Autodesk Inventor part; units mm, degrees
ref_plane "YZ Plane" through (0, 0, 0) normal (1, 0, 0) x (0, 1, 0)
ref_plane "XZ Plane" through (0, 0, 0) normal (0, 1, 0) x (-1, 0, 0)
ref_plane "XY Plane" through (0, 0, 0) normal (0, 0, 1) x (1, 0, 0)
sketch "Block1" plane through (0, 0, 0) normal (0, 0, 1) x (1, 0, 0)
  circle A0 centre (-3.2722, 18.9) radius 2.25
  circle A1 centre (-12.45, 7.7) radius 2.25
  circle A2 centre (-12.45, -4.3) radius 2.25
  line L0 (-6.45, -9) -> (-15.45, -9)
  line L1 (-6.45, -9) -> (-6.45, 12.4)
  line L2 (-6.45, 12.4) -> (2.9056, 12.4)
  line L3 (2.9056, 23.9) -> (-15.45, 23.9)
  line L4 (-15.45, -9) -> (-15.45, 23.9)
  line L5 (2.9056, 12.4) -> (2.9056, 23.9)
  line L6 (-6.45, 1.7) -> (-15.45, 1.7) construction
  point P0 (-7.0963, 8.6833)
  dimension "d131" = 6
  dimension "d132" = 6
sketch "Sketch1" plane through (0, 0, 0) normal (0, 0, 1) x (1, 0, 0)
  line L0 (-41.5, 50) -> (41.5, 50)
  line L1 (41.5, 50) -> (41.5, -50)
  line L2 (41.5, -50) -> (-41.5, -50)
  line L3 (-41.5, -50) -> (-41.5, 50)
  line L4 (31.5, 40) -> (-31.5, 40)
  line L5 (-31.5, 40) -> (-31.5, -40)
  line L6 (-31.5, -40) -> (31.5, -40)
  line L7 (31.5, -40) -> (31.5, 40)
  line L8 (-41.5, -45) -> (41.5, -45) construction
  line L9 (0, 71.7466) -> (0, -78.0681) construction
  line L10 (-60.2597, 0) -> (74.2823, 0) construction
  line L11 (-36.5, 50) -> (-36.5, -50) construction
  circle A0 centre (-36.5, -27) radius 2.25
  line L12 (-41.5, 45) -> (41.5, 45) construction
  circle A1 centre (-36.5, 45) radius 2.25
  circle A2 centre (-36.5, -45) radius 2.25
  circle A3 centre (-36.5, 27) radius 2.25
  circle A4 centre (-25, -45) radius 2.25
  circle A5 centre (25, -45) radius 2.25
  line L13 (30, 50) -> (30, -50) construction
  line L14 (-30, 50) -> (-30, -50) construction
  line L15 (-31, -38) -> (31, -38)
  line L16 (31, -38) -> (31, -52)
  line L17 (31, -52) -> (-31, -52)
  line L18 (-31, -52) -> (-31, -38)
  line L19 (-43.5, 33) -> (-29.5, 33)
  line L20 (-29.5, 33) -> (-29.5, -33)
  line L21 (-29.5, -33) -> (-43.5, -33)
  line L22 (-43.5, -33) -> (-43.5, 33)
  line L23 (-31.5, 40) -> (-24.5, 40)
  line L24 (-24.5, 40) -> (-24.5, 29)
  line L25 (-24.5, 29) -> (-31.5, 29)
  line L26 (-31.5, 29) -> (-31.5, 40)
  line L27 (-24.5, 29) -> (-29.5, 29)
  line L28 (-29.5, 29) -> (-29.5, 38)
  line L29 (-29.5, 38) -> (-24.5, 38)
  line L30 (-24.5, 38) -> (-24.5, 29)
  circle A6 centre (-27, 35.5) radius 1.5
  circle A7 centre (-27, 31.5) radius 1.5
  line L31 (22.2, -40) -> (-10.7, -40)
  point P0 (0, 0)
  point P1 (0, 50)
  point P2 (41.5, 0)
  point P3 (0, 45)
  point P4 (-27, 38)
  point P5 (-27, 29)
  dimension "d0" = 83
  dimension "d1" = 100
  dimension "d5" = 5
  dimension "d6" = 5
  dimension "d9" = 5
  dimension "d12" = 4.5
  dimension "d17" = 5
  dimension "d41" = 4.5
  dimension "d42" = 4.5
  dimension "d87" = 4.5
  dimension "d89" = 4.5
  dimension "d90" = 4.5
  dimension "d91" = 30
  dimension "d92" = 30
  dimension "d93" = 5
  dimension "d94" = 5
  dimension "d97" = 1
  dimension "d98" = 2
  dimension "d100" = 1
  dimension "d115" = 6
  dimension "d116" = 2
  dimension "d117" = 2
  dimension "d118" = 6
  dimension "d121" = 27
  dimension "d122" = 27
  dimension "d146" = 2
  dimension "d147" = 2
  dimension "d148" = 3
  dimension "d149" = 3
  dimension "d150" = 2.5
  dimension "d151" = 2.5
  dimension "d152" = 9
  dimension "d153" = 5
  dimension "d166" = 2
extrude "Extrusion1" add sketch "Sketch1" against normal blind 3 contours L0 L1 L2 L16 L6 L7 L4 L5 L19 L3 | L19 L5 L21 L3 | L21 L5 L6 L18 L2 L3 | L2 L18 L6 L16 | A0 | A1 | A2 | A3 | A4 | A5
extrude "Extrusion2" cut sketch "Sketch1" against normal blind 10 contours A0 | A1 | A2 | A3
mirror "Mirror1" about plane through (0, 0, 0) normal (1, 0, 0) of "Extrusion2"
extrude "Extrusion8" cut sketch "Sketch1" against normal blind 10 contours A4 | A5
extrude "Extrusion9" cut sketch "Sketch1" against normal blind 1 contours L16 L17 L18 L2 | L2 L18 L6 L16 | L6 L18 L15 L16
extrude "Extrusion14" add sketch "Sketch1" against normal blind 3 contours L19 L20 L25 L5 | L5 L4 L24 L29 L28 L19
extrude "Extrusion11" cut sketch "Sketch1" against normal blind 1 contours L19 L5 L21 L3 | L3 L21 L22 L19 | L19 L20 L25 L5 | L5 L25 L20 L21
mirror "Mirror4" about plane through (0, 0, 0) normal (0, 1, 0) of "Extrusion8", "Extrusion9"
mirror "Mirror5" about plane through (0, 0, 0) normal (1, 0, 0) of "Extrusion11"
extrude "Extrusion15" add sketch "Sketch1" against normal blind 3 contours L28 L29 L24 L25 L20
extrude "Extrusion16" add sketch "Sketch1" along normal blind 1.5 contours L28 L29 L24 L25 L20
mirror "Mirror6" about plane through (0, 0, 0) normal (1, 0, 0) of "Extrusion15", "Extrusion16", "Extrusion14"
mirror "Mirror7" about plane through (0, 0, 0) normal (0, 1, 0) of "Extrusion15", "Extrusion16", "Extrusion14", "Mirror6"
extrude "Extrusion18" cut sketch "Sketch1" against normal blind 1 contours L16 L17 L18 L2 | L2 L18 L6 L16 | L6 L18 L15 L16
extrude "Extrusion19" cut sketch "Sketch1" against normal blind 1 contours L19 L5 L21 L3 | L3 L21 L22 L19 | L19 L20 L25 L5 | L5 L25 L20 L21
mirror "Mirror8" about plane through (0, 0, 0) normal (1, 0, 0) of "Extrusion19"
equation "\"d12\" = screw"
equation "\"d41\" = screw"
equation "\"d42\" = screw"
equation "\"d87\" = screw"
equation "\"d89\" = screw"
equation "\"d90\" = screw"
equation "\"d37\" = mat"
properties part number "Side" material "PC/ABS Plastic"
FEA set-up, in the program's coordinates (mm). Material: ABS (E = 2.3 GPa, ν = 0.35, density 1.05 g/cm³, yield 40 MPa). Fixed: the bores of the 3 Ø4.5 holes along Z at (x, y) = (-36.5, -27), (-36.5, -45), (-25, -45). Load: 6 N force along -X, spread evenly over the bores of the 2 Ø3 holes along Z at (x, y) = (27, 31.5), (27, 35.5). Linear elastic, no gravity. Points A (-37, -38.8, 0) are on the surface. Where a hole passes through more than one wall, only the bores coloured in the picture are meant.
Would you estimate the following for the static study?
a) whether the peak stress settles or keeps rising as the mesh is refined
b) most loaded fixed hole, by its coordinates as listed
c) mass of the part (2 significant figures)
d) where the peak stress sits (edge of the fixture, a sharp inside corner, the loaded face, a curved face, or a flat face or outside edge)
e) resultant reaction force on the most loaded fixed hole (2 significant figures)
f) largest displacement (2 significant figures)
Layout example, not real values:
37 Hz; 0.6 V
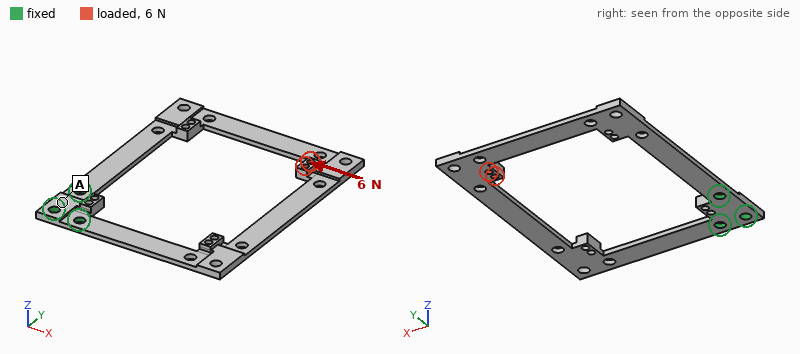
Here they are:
keeps rising; (-36.5, -27); 8.0 g; edge of the fixture; 9.8 N; 1.6 mm
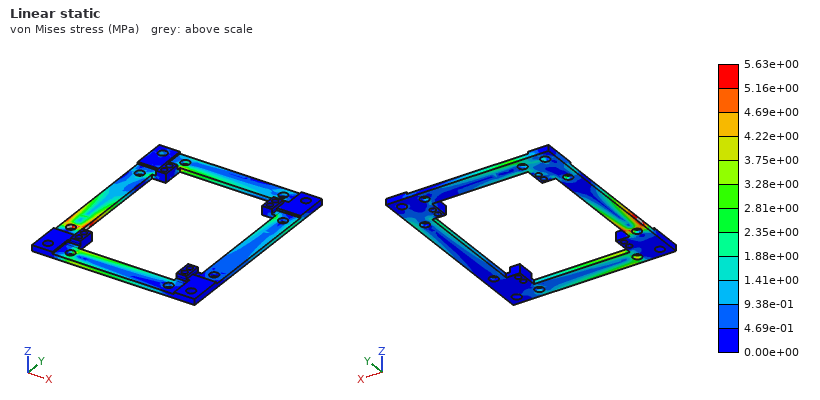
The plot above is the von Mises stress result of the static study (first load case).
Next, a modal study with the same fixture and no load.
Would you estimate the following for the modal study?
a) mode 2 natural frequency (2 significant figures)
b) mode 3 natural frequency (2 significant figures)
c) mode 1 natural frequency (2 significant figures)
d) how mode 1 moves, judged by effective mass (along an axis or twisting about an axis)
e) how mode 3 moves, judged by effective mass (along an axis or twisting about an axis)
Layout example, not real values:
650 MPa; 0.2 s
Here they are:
66 Hz; 120 Hz; 30 Hz; along Z; along Z
